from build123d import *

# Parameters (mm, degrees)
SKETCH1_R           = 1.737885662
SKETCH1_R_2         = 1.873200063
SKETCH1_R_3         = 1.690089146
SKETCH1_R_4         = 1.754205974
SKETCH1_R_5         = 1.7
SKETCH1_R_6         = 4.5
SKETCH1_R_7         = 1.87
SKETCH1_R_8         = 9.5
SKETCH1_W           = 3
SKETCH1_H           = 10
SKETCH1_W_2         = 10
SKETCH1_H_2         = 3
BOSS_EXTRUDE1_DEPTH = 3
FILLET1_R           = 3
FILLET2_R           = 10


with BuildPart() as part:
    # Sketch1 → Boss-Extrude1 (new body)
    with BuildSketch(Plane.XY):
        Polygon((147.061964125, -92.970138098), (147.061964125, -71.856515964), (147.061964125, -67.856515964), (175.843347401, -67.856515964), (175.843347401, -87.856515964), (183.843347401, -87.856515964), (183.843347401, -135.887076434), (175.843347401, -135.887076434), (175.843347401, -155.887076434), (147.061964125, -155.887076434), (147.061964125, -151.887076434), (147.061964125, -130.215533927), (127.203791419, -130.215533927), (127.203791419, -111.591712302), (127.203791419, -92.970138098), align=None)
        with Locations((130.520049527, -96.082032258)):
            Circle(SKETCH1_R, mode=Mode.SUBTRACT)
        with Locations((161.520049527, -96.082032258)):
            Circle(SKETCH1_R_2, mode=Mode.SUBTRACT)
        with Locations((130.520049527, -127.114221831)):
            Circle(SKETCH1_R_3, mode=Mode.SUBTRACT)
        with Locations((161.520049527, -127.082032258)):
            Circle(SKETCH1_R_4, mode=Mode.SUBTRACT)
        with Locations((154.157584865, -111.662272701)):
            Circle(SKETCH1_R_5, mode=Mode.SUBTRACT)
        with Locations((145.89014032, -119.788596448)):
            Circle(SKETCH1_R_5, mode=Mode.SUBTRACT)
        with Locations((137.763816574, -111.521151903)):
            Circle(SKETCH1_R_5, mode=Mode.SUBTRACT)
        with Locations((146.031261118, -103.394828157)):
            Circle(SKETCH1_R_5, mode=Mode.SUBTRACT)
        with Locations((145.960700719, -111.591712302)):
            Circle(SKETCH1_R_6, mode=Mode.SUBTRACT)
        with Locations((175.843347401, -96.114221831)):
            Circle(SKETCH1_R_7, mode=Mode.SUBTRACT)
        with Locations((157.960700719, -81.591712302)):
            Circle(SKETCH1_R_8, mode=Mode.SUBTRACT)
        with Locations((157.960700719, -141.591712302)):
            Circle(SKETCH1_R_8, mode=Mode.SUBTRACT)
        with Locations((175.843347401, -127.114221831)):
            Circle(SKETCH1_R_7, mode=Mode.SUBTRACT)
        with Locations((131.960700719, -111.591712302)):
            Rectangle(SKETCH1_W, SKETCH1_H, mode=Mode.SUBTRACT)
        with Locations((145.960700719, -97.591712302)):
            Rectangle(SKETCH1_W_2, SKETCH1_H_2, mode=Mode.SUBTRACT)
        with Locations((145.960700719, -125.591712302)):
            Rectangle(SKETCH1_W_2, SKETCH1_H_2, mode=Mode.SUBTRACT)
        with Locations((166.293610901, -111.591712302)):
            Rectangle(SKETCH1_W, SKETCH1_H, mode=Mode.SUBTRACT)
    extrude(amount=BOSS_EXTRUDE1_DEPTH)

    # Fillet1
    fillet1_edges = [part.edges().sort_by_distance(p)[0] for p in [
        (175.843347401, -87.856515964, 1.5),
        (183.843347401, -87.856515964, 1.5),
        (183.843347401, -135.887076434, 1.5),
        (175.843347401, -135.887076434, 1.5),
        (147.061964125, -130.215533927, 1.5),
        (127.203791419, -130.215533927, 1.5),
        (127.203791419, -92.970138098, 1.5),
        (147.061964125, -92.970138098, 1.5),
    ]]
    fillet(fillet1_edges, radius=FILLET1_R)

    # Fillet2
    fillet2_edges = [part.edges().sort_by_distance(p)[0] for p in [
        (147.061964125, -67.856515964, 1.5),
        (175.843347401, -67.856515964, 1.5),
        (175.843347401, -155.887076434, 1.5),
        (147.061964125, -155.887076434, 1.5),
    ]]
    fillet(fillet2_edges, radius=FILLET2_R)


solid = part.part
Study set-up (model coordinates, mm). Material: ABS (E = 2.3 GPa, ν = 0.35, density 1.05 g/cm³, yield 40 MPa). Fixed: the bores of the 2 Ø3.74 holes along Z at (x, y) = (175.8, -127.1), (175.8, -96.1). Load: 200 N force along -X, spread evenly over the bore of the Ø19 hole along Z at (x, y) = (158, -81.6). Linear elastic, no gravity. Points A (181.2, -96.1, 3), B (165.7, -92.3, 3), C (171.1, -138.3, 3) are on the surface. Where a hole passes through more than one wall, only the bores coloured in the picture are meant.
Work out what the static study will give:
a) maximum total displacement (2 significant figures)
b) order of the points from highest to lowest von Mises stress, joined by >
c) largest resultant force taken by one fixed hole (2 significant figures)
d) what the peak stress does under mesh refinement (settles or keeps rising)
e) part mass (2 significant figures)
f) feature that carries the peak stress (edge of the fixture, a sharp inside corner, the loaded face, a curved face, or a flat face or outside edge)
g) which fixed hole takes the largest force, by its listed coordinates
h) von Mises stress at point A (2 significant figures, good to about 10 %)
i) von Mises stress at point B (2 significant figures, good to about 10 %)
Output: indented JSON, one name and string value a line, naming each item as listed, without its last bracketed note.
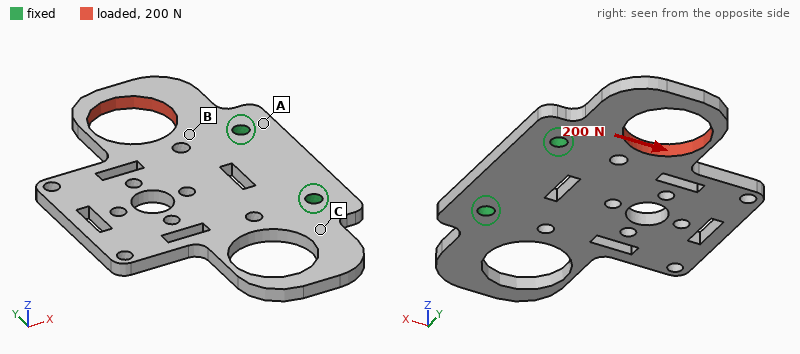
{
  "maximum total displacement": "0.59 mm",
  "order of the points from highest to lowest von Mises stress, joined by >": "B > A > C",
  "largest resultant force taken by one fixed hole": "280 N",
  "what the peak stress does under mesh refinement": "keeps rising",
  "part mass": "8.6 g",
  "feature that carries the peak stress": "a sharp inside corner",
  "which fixed hole takes the largest force, by its listed coordinates": "(175.8, -96.1)",
  "von Mises stress at point A": "5.2 MPa",
  "von Mises stress at point B": "10.0 MPa"
}
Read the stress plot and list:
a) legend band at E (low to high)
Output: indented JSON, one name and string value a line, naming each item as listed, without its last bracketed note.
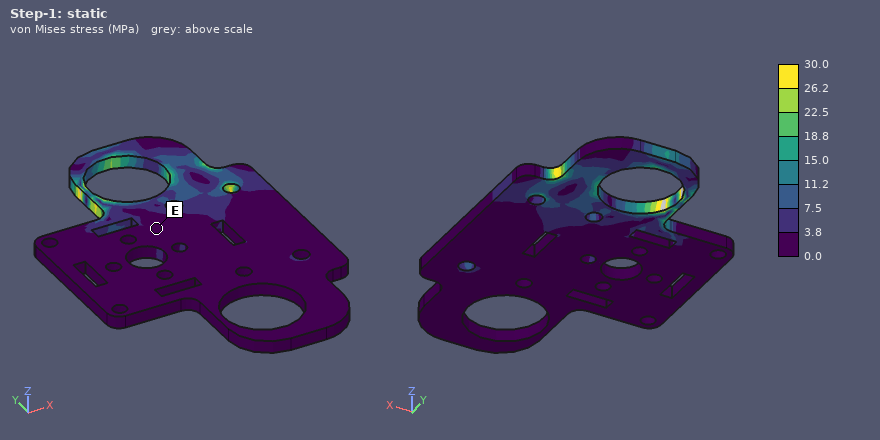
{
  "legend band at E": "0.0 to 3.8 MPa"
}
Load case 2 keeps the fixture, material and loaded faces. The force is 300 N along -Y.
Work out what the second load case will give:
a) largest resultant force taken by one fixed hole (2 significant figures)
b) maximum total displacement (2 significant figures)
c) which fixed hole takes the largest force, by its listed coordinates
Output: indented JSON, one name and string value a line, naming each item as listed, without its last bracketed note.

{
  "largest resultant force taken by one fixed hole": "240 N",
  "maximum total displacement": "0.49 mm",
  "which fixed hole takes the largest force, by its listed coordinates": "(175.8, -96.1)"
}
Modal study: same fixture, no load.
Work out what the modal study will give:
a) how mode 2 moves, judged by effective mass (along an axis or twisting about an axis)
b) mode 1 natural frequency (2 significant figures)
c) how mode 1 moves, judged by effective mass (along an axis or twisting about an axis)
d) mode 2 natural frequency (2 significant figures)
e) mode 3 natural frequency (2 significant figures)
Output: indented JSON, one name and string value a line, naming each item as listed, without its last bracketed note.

{
  "how mode 2 moves, judged by effective mass": "twisting about X",
  "mode 1 natural frequency": "340 Hz",
  "how mode 1 moves, judged by effective mass": "along Z",
  "mode 2 natural frequency": "680 Hz",
  "mode 3 natural frequency": "790 Hz"
}
